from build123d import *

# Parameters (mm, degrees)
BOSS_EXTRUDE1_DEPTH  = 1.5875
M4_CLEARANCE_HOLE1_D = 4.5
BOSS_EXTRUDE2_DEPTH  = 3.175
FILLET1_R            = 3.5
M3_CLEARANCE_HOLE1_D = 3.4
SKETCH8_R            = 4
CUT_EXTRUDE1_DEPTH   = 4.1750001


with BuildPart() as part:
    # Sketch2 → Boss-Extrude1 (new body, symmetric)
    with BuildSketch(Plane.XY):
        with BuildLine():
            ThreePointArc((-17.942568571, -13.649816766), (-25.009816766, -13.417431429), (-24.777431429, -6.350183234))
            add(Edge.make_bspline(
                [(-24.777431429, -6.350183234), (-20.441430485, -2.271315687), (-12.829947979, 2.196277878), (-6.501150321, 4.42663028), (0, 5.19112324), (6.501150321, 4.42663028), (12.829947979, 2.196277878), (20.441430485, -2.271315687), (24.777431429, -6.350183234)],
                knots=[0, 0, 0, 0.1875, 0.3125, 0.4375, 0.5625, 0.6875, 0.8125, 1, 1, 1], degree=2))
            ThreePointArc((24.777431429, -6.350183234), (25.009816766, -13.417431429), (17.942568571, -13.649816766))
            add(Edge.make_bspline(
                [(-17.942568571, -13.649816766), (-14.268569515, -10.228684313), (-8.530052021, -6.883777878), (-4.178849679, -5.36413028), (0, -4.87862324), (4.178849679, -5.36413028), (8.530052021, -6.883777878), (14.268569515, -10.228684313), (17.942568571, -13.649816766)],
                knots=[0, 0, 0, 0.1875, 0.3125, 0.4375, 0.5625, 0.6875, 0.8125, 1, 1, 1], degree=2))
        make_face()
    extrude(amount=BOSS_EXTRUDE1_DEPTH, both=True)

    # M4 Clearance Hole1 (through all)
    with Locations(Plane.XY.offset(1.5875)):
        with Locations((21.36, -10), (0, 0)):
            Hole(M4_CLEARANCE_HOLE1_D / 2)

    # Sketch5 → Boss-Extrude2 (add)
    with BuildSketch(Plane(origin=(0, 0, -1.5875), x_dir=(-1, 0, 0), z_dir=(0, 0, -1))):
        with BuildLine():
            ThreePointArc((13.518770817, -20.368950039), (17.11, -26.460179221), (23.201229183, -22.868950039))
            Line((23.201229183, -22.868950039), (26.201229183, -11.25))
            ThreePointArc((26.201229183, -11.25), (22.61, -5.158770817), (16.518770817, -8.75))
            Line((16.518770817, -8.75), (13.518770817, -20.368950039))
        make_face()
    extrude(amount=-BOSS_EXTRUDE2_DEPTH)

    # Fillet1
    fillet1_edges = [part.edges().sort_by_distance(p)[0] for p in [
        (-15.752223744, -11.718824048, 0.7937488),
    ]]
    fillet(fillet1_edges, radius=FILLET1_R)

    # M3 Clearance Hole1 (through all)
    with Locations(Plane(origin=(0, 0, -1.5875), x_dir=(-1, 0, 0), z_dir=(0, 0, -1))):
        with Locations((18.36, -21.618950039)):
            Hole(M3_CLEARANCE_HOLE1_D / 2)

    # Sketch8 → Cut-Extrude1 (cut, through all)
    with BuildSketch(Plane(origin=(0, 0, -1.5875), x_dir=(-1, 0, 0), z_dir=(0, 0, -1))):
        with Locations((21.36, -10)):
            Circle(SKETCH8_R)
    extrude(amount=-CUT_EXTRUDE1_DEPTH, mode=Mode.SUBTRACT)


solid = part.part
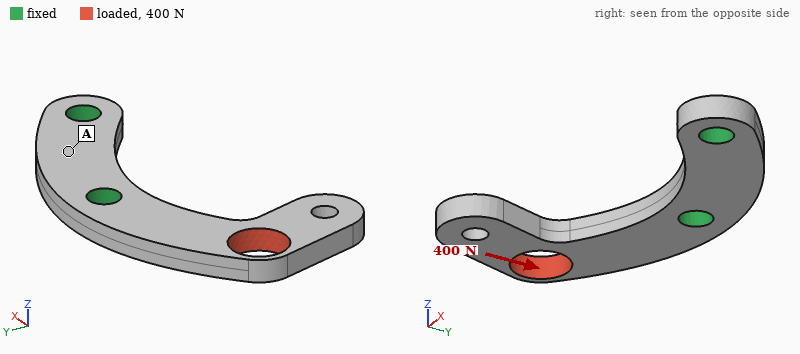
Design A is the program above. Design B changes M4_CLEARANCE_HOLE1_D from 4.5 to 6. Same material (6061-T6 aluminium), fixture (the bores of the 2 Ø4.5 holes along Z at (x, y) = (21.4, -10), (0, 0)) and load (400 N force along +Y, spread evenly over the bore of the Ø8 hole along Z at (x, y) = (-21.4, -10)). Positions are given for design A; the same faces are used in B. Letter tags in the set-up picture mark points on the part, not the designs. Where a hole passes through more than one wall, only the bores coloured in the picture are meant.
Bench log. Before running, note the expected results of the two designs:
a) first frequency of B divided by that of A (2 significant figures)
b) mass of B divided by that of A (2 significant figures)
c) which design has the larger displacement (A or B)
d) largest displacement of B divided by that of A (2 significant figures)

1.0
0.96
A
0.89
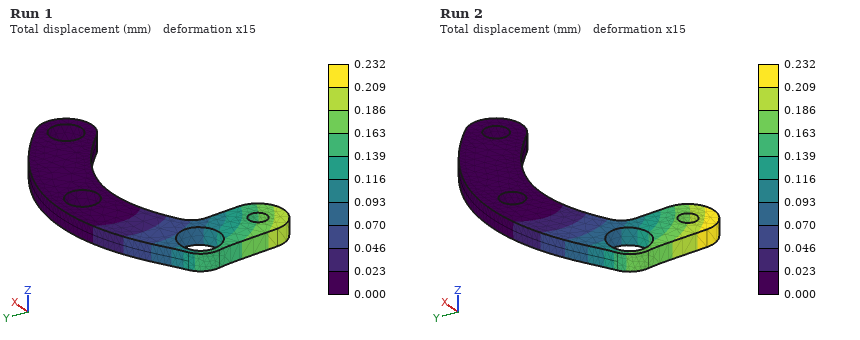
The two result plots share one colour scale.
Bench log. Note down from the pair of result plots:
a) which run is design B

Run 1
